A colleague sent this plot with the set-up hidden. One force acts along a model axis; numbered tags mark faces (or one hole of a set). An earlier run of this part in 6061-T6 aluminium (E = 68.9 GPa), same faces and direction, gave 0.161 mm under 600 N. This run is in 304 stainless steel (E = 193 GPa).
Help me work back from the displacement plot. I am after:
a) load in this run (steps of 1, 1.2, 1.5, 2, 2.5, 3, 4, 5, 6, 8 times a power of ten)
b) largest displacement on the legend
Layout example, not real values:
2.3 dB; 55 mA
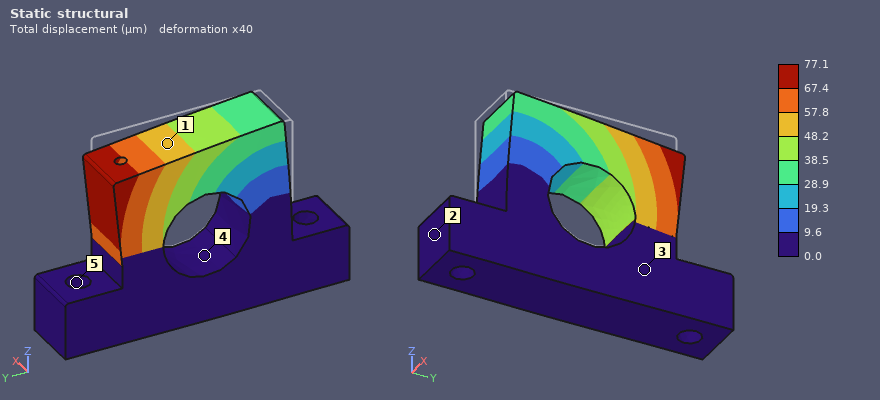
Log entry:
800 N; 77.1 µm
